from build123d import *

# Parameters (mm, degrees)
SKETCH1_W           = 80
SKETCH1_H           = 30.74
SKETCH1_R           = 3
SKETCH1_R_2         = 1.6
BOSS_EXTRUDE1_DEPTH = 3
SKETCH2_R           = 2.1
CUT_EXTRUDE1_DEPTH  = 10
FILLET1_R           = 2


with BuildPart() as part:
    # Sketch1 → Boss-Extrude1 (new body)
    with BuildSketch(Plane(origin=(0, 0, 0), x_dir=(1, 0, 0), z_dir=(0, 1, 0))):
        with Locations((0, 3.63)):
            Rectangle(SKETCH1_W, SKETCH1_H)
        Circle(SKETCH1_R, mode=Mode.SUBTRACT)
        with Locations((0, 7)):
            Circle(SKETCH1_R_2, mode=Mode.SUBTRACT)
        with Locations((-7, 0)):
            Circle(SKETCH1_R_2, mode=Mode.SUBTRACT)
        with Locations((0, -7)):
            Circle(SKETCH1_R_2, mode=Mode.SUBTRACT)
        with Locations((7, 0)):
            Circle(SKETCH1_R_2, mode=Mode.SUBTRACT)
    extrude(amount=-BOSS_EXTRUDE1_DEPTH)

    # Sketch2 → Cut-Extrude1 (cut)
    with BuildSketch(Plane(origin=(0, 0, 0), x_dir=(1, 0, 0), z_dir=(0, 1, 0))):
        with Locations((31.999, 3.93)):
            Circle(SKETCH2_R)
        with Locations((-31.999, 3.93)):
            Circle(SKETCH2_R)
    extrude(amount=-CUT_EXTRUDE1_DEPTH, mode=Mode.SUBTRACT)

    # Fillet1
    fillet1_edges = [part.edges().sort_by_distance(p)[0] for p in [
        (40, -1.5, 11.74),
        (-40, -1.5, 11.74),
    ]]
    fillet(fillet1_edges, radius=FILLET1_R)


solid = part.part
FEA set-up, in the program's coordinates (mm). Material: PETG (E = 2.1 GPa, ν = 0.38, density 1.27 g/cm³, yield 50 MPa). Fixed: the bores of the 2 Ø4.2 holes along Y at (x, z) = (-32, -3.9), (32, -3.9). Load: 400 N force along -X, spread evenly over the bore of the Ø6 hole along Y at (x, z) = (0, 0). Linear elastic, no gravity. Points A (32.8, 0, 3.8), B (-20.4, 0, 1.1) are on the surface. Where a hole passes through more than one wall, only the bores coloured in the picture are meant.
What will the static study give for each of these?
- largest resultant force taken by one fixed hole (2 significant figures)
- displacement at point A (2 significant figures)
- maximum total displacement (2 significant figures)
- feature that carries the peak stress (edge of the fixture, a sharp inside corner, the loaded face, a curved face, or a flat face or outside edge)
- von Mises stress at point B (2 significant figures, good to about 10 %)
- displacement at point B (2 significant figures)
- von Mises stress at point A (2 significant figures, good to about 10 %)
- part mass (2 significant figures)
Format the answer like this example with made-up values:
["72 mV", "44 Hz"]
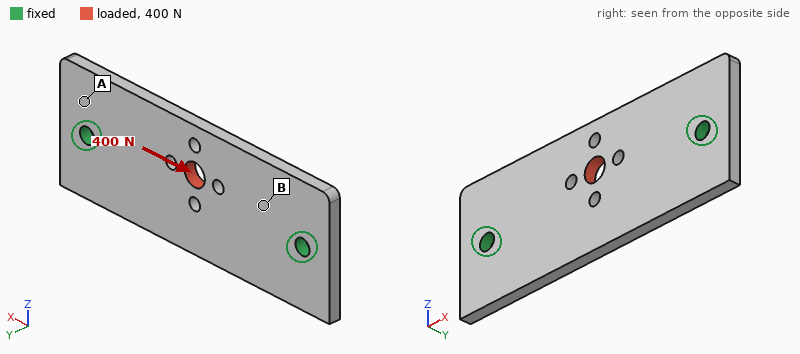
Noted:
["200 N", "19 µm", "76 µm", "a curved face", "3.6 MPa", "27 µm", "1.5 MPa", "9.0 g"]
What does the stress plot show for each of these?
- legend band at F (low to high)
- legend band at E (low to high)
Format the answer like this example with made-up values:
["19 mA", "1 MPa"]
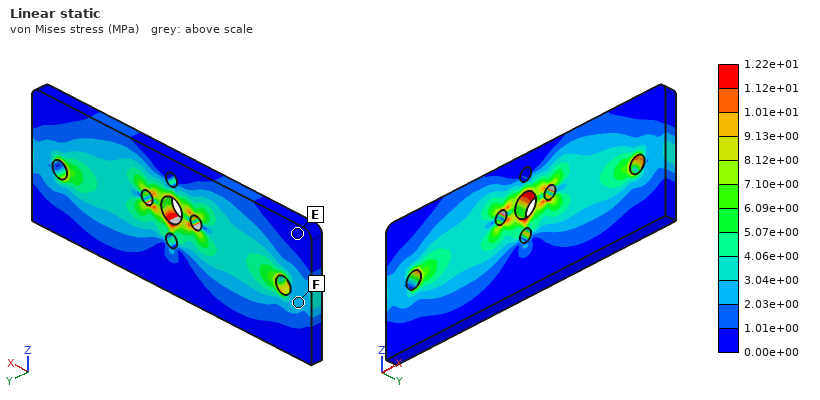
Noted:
["2.03e+00 to 3.04e+00 MPa", "0.00e+00 to 1.01e+00 MPa"]
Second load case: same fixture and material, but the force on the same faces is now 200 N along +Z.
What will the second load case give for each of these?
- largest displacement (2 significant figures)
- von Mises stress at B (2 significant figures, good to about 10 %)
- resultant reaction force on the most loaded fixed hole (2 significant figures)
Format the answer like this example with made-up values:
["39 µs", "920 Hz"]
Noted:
["0.13 mm", "2.6 MPa", "100 N"]
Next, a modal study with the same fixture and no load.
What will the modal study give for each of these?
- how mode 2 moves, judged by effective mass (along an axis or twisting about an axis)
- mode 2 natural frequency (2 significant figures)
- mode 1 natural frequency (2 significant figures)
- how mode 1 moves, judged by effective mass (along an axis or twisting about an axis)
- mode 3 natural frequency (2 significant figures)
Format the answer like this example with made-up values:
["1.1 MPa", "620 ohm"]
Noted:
["twisting about X", "1200 Hz", "900 Hz", "along Y", "2200 Hz"]
